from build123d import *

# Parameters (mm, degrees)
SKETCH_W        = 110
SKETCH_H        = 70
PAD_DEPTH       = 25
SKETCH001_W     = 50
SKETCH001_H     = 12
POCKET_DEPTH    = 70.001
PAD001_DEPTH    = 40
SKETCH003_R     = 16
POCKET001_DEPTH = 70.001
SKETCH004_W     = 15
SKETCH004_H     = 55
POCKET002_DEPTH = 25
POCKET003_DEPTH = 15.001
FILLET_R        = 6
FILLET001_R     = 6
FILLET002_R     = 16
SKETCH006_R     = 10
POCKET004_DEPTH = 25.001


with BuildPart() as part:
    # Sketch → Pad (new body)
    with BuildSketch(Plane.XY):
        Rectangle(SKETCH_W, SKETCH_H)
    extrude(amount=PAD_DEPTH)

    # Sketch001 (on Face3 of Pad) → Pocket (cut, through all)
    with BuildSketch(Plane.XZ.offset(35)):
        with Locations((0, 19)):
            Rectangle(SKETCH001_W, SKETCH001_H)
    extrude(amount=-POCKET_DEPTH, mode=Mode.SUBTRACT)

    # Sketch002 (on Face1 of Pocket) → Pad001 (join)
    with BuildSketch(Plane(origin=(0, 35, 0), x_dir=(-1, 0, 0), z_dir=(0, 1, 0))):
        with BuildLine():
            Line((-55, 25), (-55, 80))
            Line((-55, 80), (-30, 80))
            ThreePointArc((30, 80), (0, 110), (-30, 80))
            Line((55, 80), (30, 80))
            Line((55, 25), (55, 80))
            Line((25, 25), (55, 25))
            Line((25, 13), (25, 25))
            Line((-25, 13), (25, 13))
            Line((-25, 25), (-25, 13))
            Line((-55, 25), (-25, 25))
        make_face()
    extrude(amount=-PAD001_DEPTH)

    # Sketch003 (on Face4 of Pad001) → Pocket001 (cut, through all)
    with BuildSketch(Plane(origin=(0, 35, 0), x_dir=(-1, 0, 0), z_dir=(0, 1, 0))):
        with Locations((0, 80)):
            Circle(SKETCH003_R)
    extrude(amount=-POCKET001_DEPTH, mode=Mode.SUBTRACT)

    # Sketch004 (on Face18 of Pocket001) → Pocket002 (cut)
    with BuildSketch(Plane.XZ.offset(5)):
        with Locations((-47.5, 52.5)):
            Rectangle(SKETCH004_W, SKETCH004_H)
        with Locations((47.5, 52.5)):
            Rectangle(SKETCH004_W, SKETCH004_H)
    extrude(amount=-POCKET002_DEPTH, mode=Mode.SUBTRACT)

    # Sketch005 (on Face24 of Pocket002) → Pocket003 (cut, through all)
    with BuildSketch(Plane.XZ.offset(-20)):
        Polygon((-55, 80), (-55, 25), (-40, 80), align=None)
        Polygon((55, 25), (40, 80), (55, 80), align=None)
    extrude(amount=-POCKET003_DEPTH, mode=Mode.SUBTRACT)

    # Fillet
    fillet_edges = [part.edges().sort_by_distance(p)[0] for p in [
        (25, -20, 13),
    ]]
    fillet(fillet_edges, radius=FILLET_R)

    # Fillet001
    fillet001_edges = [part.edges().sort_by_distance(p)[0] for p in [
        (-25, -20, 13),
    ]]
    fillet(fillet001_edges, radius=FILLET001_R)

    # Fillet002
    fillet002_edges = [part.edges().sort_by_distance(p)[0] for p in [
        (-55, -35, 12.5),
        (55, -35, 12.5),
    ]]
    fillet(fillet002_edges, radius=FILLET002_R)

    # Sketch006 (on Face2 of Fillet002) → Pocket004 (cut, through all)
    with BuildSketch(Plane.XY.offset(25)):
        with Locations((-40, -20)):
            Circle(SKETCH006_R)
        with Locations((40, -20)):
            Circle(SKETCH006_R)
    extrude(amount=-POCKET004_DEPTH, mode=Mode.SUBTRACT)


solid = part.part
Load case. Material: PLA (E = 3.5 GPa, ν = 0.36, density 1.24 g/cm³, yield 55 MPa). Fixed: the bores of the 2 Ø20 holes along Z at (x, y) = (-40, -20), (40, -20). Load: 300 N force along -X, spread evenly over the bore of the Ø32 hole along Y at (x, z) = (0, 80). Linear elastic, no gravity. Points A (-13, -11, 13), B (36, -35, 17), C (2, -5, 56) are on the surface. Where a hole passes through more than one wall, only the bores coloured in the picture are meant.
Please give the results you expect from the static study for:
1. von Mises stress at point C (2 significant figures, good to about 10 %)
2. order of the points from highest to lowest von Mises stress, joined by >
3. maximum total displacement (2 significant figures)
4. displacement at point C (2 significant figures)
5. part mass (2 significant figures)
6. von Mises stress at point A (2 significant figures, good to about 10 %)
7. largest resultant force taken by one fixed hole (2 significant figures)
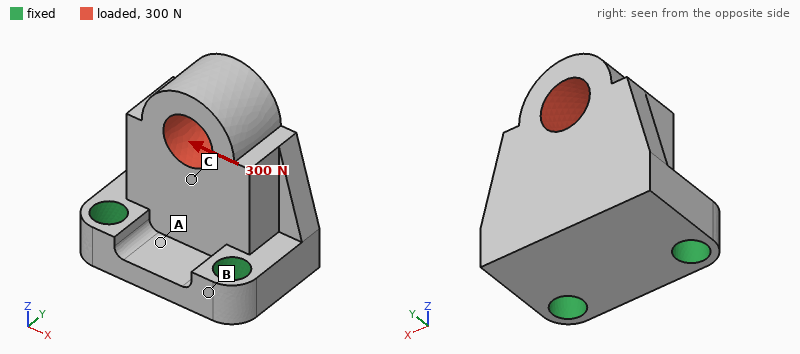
0.51 MPa
C > A > B
36 µm
16 µm
460 g
0.27 MPa
300 N
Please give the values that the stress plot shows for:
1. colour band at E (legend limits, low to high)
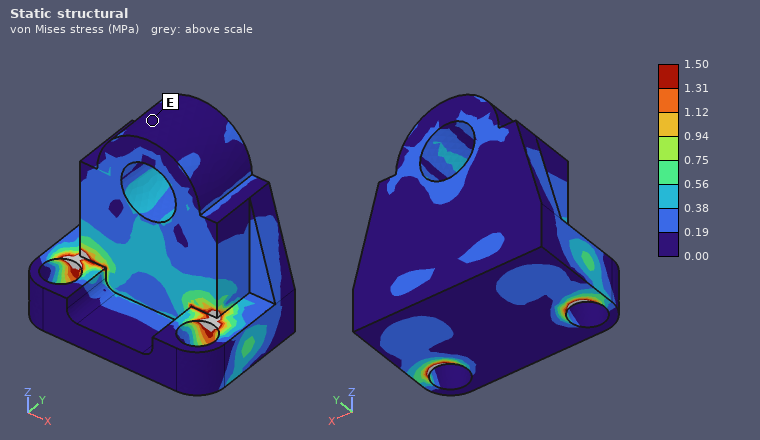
0.00 to 0.19 MPa
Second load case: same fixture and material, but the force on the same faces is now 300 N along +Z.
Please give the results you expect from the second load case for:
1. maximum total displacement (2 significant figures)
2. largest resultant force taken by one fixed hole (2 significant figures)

43 µm
150 N
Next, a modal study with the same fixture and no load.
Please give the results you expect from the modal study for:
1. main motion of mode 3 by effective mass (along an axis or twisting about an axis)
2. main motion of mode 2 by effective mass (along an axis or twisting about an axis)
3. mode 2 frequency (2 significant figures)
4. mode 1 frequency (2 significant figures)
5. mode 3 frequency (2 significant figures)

along Z
along X
1300 Hz
620 Hz
2100 Hz
